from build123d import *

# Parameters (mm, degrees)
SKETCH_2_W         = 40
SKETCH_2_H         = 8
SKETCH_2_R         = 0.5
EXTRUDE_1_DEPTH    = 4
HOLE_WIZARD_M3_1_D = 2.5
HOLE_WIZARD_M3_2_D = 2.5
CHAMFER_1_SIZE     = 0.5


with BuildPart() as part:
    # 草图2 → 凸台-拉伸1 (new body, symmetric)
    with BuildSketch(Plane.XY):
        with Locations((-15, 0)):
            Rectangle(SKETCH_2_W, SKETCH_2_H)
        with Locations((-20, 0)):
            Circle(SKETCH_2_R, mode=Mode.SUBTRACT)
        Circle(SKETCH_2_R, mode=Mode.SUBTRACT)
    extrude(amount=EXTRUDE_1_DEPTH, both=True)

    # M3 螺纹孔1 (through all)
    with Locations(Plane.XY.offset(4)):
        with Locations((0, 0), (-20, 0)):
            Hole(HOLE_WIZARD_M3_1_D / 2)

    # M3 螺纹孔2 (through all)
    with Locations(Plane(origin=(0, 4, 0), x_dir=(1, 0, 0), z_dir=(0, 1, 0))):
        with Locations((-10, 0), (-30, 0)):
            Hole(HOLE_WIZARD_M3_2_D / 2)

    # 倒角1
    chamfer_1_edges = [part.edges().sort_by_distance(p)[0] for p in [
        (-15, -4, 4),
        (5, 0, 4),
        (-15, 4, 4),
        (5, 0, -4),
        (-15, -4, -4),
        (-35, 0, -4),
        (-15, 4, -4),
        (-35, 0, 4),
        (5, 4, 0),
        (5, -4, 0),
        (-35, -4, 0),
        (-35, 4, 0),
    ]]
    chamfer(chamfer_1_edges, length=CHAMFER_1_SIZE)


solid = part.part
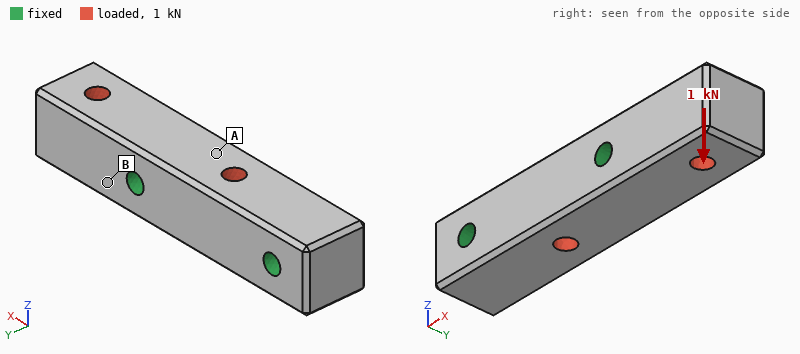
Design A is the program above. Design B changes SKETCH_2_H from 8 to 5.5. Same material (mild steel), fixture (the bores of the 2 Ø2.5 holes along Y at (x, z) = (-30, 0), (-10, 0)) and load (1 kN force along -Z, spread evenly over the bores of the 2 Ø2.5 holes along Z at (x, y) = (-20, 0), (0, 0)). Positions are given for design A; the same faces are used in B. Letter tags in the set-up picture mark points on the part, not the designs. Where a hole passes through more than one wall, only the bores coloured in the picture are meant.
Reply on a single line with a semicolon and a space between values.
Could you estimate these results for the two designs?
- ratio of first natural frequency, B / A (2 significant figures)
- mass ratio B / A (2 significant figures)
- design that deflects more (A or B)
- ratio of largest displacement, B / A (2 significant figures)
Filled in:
0.93; 0.67; B; 1.5
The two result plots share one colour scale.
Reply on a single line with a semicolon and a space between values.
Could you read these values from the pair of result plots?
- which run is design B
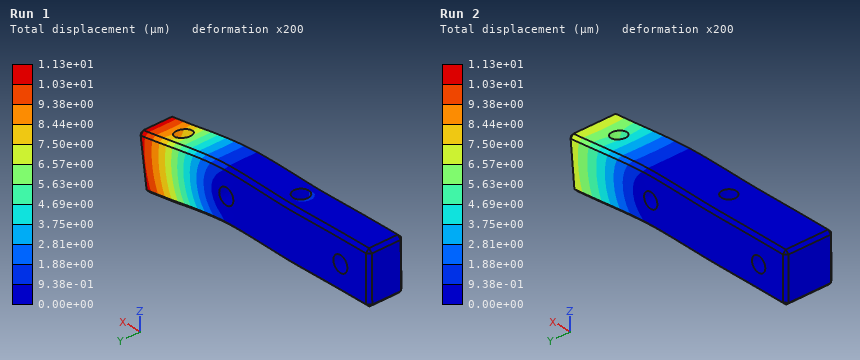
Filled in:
Run 1
